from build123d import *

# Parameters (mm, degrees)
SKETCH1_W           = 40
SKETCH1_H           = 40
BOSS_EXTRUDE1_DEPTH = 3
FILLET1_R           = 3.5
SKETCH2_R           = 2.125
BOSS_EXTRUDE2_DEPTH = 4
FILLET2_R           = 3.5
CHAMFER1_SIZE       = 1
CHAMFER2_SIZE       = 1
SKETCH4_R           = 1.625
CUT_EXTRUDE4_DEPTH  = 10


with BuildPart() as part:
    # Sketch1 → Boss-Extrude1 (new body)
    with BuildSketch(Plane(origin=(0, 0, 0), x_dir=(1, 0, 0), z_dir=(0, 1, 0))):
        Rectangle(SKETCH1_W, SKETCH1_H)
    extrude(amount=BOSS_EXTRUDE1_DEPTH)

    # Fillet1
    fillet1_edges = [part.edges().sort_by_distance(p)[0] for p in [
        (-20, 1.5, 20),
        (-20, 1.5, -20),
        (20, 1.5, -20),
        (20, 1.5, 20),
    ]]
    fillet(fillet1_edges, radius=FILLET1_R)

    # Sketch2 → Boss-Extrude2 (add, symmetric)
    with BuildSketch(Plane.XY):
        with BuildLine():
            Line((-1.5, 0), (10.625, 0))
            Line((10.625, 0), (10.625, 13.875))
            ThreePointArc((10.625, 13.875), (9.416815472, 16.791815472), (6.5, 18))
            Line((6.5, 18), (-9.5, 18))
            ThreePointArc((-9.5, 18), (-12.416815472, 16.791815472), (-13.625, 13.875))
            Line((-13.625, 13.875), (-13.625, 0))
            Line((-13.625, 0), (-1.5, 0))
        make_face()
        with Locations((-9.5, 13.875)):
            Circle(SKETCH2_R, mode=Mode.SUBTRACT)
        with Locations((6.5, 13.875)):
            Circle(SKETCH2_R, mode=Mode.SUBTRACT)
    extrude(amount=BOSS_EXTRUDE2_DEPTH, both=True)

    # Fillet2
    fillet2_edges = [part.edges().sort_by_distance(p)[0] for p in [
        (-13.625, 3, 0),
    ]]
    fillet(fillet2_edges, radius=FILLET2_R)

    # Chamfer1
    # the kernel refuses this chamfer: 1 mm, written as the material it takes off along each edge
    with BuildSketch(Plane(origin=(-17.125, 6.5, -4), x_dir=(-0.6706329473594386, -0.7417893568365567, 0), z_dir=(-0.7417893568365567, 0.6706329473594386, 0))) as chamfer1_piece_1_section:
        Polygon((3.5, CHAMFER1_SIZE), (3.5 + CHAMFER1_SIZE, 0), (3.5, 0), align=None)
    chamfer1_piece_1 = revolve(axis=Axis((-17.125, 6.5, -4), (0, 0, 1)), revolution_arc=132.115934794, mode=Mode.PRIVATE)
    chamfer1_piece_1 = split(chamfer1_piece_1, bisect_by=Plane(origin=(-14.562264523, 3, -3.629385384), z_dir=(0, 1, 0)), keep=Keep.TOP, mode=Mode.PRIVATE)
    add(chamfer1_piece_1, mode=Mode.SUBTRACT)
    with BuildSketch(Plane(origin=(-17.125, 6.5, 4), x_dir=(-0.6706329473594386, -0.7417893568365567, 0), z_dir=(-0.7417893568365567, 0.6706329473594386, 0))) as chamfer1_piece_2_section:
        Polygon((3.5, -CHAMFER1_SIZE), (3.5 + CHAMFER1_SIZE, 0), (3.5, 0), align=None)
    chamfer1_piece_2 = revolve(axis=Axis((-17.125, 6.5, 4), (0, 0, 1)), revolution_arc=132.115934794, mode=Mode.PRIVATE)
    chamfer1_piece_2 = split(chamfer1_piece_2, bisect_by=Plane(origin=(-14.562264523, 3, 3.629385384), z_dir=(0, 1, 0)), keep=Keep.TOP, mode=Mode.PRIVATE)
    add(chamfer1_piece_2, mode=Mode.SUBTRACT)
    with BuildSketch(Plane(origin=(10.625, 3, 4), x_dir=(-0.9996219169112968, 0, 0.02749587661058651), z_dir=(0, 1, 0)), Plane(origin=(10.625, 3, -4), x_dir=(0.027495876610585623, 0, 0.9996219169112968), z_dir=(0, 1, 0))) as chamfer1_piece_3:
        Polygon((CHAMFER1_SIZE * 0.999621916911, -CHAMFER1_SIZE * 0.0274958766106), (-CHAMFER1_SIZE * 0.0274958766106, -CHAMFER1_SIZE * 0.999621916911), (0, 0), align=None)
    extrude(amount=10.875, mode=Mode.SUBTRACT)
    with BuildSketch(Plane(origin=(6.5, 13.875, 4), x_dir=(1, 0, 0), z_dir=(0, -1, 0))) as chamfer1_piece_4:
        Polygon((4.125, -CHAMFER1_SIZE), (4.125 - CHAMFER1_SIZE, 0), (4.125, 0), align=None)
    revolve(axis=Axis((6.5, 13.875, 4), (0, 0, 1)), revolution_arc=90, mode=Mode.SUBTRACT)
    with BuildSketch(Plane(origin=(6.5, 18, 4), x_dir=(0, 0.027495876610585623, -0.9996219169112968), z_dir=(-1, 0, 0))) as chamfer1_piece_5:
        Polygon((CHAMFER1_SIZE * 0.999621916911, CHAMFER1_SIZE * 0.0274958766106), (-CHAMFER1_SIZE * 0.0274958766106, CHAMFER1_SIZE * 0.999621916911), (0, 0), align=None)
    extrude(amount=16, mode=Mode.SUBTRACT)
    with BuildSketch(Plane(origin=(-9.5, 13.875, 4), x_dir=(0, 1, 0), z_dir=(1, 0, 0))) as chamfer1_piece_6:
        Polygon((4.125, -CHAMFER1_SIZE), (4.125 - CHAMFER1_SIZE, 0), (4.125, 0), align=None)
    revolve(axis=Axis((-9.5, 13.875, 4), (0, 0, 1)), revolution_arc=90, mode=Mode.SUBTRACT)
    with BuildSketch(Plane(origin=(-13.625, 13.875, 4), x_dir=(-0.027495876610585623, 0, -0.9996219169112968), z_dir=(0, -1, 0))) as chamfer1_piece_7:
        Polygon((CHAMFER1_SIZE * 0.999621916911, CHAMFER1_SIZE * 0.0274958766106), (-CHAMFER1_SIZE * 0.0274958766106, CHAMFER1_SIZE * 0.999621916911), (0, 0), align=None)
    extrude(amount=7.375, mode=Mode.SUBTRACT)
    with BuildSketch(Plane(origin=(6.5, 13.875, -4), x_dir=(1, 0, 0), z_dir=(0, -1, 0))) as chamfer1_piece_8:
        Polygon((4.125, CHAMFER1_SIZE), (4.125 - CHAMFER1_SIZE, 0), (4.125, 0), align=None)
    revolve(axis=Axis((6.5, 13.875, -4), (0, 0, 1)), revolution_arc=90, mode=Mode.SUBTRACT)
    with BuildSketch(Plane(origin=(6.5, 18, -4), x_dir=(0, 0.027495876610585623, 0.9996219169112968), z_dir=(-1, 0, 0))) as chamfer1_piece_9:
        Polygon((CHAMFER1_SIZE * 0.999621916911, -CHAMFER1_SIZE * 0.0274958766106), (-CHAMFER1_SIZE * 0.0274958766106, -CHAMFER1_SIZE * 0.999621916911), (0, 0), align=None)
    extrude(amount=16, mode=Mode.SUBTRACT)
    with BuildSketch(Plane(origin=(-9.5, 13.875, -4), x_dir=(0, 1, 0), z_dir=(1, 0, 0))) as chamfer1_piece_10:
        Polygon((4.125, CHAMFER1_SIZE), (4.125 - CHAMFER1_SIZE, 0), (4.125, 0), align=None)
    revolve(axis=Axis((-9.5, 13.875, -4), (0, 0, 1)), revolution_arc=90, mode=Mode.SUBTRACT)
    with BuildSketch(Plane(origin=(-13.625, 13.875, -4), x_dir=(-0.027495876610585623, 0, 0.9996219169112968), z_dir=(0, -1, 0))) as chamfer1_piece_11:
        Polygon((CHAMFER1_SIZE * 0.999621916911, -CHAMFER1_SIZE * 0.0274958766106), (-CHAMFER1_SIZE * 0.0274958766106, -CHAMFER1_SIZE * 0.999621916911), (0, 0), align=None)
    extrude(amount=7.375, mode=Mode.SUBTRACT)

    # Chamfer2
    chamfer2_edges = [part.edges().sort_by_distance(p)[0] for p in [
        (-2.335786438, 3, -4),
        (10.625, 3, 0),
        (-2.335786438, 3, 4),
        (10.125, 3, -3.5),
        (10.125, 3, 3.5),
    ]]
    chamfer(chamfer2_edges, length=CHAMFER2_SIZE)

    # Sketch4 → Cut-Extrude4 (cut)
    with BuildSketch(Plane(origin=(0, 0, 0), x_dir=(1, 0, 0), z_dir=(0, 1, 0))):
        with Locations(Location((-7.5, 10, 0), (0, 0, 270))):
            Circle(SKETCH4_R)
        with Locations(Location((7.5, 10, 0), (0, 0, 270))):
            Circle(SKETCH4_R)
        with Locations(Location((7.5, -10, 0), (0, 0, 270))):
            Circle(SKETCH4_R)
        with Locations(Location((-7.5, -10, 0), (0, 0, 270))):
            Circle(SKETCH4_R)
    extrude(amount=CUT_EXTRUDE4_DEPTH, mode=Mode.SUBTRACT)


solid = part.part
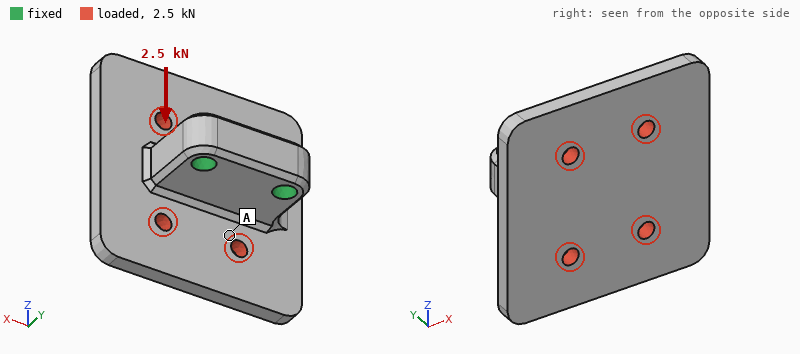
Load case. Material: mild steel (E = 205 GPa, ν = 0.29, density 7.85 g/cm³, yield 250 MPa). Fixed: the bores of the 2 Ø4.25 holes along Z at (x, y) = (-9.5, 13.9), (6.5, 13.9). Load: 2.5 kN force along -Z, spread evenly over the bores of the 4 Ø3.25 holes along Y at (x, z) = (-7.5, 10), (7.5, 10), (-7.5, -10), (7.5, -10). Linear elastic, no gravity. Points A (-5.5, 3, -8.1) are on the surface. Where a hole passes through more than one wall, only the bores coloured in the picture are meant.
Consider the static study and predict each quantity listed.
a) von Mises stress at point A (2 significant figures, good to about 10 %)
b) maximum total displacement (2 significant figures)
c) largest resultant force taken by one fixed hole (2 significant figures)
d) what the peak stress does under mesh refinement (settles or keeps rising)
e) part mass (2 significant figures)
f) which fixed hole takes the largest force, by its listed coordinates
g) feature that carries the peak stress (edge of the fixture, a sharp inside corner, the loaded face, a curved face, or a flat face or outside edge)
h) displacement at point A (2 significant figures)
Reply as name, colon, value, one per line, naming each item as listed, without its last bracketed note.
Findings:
von Mises stress at point A: 21 MPa
maximum total displacement: 24 µm
largest resultant force taken by one fixed hole: 1.4 kN
what the peak stress does under mesh refinement: keeps rising
part mass: 57 g
which fixed hole takes the largest force, by its listed coordinates: (6.5, 13.9)
feature that carries the peak stress: edge of the fixture
displacement at point A: 11 µm
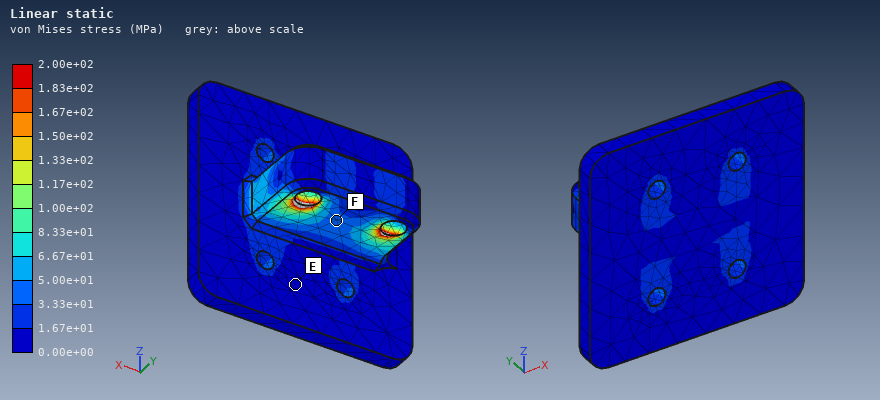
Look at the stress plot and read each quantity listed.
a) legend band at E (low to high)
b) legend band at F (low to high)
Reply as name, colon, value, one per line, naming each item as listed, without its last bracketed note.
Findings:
legend band at E: 0.00e+00 to 1.67e+01 MPa
legend band at F: 3.33e+01 to 5.00e+01 MPa
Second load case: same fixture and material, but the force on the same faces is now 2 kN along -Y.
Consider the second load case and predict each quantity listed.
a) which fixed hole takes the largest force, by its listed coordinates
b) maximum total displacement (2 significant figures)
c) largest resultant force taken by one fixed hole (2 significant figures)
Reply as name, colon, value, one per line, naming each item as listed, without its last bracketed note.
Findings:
which fixed hole takes the largest force, by its listed coordinates: (6.5, 13.9)
maximum total displacement: 24 µm
largest resultant force taken by one fixed hole: 1.2 kN
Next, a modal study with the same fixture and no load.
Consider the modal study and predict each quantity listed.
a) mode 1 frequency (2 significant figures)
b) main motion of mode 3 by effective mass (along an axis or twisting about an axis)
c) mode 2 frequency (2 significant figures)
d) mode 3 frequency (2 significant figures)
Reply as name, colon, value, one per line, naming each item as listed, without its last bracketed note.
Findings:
mode 1 frequency: 6000 Hz
main motion of mode 3 by effective mass: twisting about Y
mode 2 frequency: 8000 Hz
mode 3 frequency: 8300 Hz
